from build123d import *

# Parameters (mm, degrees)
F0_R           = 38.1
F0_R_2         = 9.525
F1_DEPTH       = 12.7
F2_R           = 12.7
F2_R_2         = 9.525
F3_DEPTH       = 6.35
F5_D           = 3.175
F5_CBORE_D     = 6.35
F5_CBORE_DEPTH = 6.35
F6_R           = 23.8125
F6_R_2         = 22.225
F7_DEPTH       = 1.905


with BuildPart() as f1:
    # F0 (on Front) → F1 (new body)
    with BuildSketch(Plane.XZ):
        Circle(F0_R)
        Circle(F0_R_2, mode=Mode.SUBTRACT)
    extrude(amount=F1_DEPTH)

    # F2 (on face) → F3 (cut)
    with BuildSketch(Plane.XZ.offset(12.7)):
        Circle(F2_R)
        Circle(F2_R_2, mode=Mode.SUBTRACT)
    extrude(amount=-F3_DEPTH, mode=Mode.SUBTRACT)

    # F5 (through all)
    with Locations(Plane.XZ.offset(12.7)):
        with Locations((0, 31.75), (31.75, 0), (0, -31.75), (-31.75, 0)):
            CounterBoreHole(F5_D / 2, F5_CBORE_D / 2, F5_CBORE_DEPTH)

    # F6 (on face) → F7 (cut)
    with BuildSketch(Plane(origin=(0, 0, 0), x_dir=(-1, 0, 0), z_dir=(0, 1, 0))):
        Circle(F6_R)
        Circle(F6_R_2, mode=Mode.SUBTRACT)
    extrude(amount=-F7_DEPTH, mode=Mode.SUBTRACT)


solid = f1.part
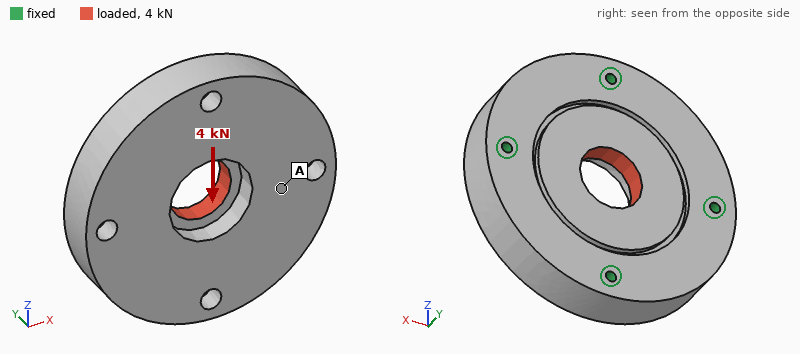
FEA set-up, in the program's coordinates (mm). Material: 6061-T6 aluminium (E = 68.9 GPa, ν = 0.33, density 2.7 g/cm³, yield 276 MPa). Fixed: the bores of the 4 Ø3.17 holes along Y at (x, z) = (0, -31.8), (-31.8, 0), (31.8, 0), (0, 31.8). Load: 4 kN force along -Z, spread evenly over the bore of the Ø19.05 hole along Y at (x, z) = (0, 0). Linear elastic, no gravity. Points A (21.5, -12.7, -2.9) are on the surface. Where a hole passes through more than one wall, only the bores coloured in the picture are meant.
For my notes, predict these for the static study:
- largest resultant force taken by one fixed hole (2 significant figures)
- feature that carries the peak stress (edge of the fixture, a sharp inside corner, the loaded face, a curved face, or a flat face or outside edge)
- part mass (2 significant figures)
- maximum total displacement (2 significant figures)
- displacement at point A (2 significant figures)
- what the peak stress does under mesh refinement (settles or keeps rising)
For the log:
1.1 kN
edge of the fixture
140 g
4.3 µm
1.7 µm
keeps rising
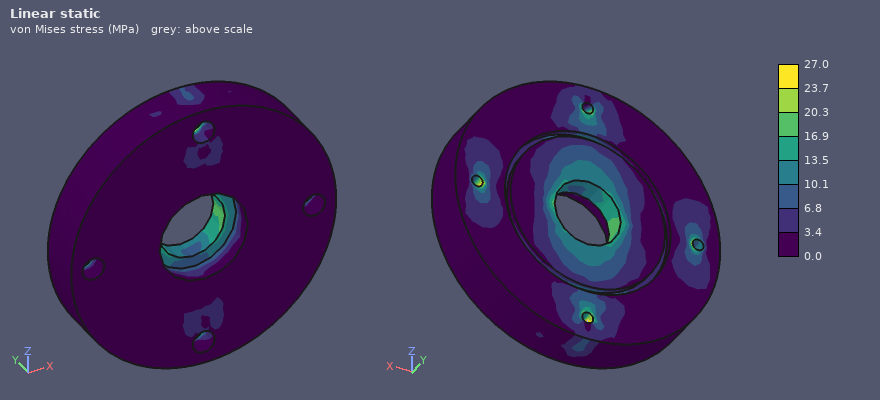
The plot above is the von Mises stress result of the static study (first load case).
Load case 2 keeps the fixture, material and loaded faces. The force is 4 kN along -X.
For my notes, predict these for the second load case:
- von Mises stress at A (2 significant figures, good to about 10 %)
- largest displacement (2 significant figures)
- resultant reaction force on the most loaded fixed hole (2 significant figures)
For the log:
3.4 MPa
4.3 µm
1.1 kN
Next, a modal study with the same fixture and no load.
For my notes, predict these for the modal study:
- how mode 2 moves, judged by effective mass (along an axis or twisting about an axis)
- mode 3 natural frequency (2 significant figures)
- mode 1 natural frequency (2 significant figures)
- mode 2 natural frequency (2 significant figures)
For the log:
along Y
14 kHz
12 kHz
13 kHz
